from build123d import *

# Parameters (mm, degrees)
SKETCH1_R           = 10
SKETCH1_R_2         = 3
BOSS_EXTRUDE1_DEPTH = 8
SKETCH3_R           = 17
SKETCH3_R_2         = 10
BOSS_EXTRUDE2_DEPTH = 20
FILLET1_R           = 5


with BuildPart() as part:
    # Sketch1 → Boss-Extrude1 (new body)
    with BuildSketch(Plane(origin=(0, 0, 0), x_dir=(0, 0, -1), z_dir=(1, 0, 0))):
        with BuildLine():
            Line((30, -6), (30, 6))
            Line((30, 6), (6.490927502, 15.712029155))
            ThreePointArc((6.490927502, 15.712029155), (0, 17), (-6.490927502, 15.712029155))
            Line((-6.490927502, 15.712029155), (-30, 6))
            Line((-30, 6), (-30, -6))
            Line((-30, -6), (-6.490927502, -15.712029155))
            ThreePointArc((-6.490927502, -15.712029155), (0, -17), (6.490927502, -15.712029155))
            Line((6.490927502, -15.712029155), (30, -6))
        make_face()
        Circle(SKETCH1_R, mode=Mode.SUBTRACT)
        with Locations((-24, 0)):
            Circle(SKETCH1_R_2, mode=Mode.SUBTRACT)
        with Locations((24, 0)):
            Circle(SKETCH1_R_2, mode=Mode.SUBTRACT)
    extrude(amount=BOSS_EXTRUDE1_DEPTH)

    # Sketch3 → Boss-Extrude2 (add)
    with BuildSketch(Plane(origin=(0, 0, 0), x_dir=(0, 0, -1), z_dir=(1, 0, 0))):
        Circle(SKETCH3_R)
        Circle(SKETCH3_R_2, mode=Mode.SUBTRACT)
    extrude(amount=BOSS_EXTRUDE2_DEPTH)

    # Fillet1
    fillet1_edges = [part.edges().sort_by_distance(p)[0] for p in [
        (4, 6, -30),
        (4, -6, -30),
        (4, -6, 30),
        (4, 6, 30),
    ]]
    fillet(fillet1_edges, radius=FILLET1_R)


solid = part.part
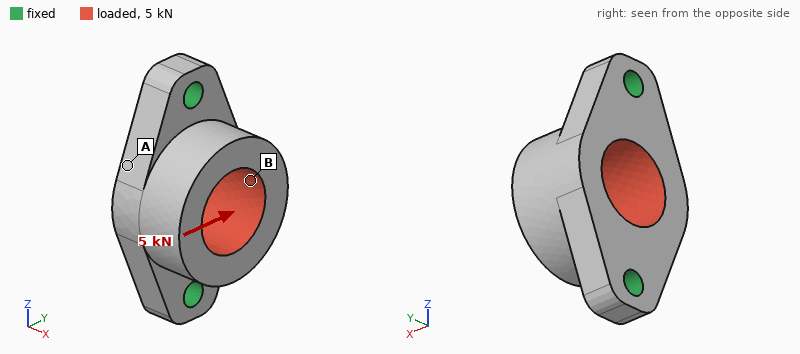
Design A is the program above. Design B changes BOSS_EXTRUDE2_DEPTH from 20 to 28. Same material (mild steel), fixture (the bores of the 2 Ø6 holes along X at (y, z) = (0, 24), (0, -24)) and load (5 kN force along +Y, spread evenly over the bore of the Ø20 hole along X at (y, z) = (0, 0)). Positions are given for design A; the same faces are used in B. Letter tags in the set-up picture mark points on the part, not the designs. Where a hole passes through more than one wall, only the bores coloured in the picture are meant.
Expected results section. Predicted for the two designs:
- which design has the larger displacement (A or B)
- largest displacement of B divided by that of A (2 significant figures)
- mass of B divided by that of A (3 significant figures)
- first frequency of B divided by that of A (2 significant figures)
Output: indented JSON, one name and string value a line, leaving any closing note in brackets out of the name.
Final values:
{
  "which design has the larger displacement": "B",
  "largest displacement of B divided by that of A": "1.9",
  "mass of B divided by that of A": "1.30",
  "first frequency of B divided by that of A": "0.68"
}
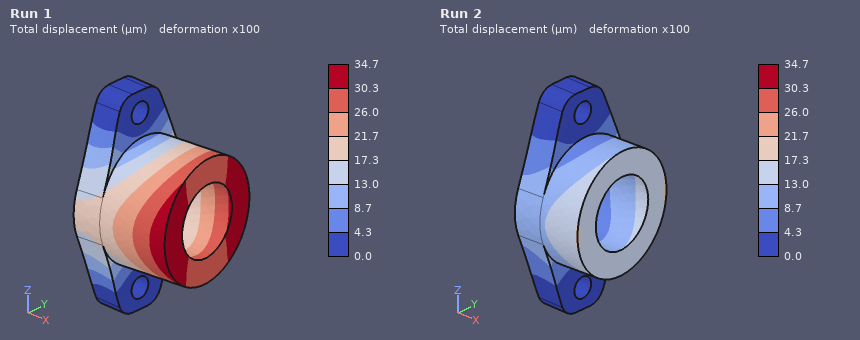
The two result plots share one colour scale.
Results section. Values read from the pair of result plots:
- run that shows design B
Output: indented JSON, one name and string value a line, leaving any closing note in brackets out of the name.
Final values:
{
  "run that shows design B": "Run 1"
}
